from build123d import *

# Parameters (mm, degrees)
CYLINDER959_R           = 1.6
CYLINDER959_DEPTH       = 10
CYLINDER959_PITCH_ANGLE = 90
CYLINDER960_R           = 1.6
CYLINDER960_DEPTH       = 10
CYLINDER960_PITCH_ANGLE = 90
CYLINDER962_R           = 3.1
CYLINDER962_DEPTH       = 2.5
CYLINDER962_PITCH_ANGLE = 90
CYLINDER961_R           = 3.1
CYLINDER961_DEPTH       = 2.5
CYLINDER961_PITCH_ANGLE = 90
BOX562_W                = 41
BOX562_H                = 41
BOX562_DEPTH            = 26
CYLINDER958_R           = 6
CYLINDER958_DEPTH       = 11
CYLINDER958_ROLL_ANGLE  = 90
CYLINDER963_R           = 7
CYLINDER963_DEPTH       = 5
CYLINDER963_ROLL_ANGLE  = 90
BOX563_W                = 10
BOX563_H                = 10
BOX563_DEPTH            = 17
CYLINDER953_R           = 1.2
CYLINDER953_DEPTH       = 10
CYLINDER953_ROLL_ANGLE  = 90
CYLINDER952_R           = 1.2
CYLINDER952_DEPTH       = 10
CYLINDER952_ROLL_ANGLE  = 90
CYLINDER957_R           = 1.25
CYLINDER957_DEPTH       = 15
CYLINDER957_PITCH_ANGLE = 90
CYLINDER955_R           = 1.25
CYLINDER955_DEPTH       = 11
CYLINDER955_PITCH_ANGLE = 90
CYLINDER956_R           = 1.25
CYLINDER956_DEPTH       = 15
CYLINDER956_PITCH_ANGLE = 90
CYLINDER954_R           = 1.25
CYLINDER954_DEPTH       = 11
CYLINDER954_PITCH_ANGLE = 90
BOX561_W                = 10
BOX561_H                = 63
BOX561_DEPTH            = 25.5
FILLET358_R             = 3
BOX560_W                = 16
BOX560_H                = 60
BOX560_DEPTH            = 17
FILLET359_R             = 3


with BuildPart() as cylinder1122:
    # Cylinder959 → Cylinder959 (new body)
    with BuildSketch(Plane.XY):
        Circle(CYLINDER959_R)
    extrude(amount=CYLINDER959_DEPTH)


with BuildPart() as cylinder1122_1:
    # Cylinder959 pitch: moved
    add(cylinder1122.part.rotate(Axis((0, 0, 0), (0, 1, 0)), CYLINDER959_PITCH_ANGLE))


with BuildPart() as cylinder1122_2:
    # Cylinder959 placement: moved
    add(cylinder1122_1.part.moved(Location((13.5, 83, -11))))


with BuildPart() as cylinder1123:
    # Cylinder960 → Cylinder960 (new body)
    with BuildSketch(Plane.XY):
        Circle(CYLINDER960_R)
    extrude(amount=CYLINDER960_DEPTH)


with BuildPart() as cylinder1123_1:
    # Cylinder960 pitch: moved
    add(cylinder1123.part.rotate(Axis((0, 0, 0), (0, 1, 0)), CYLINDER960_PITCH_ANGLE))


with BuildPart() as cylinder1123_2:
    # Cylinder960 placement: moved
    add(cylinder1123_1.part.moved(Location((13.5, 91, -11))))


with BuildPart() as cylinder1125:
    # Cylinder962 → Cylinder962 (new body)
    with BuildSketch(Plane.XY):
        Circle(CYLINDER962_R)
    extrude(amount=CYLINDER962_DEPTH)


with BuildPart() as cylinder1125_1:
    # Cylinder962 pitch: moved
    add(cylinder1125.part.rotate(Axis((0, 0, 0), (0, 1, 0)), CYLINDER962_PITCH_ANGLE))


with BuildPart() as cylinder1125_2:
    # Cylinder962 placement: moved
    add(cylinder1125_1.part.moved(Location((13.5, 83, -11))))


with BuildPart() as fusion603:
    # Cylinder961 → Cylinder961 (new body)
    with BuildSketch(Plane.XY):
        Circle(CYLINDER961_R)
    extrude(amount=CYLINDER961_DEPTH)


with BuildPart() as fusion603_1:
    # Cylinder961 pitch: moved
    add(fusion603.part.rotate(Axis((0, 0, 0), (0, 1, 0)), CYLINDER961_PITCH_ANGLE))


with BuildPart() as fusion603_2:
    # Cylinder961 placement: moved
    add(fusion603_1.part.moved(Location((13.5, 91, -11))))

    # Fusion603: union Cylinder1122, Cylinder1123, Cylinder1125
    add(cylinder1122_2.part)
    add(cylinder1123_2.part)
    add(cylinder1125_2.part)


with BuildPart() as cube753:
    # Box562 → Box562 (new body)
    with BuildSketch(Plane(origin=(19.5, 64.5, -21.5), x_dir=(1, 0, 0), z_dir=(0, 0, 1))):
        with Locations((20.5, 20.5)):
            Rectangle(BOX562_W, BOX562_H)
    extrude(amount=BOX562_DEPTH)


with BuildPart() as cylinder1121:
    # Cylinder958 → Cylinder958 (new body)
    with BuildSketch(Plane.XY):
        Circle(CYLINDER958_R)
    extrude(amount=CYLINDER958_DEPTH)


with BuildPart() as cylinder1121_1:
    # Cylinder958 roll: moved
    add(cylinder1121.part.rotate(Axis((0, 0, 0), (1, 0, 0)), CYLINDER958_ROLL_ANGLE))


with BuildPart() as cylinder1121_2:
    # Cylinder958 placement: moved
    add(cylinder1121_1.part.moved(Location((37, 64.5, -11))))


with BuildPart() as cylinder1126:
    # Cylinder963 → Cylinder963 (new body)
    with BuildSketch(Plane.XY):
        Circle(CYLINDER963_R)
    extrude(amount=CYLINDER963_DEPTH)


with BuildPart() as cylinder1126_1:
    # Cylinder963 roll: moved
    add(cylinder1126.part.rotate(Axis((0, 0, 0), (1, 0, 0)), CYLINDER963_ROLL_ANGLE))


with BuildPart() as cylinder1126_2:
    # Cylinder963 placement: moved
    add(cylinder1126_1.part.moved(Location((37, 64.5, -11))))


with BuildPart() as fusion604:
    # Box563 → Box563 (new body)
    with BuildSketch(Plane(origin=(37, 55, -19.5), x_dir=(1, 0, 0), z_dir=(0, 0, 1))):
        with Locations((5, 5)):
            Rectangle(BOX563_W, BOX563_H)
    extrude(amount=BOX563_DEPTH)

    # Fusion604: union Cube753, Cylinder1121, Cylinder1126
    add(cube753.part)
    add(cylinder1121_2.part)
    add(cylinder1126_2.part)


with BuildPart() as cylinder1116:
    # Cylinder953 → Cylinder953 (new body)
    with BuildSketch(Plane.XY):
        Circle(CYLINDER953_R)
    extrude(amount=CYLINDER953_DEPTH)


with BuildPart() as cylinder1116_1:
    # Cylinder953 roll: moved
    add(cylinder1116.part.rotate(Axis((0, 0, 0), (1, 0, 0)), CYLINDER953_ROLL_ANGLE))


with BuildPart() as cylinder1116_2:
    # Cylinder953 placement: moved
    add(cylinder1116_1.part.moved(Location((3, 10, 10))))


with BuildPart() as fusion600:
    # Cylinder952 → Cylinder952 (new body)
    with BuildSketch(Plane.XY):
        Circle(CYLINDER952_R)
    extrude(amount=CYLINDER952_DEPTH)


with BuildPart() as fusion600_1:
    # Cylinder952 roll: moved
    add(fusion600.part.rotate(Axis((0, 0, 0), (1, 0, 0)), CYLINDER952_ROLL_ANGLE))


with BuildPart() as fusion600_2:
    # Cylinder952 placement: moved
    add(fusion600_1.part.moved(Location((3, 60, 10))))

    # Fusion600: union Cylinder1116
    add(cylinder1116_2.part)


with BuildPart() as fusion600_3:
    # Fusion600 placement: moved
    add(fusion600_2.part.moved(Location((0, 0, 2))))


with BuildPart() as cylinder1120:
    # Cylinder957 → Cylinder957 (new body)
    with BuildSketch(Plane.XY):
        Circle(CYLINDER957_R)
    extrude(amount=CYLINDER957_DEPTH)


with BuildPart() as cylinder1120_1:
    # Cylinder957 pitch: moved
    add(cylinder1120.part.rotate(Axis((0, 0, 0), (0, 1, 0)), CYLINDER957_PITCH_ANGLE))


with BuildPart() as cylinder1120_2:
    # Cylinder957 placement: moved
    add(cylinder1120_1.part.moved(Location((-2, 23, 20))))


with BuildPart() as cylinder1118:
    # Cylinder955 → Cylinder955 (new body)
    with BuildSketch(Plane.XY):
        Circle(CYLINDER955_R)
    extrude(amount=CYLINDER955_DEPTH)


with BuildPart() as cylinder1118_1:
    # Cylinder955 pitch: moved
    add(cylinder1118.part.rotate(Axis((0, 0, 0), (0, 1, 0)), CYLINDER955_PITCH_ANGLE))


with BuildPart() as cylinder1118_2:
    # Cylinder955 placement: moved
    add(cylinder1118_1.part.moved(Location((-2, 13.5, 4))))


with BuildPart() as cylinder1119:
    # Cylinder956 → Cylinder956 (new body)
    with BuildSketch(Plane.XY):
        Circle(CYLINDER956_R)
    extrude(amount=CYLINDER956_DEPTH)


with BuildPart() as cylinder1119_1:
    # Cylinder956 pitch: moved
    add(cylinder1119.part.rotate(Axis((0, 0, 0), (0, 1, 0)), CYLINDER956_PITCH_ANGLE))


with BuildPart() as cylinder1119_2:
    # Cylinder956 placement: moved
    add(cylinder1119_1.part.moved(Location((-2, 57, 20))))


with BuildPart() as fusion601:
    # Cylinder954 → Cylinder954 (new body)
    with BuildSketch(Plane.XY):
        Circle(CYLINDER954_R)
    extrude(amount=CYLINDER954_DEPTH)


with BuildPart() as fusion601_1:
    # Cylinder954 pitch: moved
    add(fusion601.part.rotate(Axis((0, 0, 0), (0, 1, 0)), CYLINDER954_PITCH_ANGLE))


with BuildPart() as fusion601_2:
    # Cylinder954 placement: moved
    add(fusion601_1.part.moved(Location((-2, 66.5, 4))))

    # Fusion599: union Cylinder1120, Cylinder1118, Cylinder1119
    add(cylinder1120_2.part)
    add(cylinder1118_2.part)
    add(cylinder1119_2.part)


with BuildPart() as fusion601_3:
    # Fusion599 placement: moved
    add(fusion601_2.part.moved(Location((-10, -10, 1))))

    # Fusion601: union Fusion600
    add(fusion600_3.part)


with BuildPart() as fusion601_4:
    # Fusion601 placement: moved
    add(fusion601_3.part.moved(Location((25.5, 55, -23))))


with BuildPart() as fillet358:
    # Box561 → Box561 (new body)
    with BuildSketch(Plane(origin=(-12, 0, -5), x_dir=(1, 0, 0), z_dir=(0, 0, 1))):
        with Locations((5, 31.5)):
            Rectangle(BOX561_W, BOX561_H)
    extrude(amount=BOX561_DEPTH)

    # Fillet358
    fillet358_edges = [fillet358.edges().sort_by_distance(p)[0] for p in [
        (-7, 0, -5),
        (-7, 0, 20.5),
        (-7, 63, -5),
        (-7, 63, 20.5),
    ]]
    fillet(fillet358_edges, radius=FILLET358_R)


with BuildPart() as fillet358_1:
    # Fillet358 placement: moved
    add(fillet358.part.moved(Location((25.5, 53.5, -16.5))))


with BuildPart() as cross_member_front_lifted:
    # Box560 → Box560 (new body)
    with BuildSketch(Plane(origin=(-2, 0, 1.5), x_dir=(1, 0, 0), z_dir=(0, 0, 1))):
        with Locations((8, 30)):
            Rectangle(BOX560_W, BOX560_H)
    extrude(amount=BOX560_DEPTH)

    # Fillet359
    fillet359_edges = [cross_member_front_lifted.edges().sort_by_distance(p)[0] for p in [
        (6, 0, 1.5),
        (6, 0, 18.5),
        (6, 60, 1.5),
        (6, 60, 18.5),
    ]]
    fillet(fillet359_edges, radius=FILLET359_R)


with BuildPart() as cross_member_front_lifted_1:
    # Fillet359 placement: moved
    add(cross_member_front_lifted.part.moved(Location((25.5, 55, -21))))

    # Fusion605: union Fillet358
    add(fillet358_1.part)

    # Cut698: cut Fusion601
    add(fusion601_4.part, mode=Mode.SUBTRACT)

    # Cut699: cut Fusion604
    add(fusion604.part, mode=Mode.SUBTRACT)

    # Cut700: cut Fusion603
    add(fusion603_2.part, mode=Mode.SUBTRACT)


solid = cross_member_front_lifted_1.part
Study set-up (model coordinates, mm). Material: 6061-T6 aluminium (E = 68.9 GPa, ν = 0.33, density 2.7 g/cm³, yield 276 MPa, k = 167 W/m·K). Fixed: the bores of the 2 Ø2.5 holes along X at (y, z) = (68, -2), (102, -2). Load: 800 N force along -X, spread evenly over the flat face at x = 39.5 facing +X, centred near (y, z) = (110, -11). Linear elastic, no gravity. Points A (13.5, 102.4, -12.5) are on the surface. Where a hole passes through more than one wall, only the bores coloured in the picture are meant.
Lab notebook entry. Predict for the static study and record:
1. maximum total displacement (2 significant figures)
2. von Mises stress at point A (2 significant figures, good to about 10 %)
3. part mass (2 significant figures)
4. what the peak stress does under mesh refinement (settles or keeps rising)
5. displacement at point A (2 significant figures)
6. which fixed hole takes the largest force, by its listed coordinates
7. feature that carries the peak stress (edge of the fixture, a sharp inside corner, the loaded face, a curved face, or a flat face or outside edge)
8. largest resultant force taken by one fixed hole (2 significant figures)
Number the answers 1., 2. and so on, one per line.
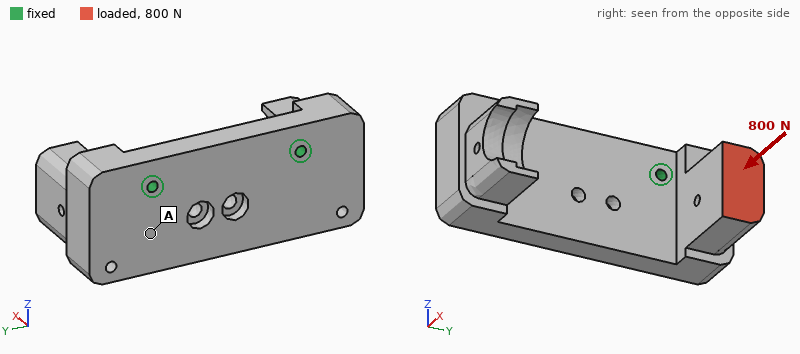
1. 75 µm
2. 19 MPa
3. 41 g
4. keeps rising
5. 19 µm
6. (102, -2)
7. edge of the fixture
8. 870 N
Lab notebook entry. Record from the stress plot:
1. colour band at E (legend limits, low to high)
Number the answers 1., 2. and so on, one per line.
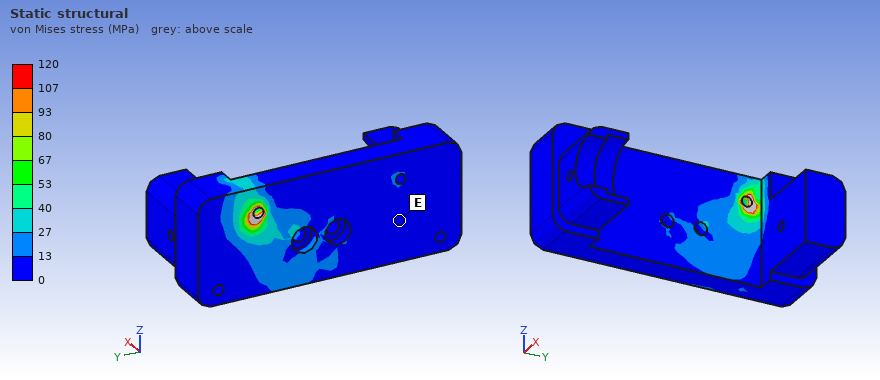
1. 0 to 13 MPa
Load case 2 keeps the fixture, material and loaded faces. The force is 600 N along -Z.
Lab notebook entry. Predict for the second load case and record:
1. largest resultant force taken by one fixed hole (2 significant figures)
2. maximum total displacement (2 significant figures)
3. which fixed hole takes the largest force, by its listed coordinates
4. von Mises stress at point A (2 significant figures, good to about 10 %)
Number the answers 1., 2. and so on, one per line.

1. 730 N
2. 0.11 mm
3. (102, -2)
4. 23 MPa
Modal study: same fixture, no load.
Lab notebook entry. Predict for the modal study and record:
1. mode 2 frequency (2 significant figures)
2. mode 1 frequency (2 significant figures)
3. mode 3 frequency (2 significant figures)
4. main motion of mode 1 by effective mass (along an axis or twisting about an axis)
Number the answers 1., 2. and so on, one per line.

1. 5800 Hz
2. 4700 Hz
3. 6300 Hz
4. along X
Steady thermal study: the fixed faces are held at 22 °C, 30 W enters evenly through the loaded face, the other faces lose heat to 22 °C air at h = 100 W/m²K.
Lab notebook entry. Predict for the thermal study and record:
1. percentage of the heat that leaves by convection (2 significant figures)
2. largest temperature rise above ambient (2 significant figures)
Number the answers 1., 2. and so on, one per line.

1. 15 %
2. 35 K
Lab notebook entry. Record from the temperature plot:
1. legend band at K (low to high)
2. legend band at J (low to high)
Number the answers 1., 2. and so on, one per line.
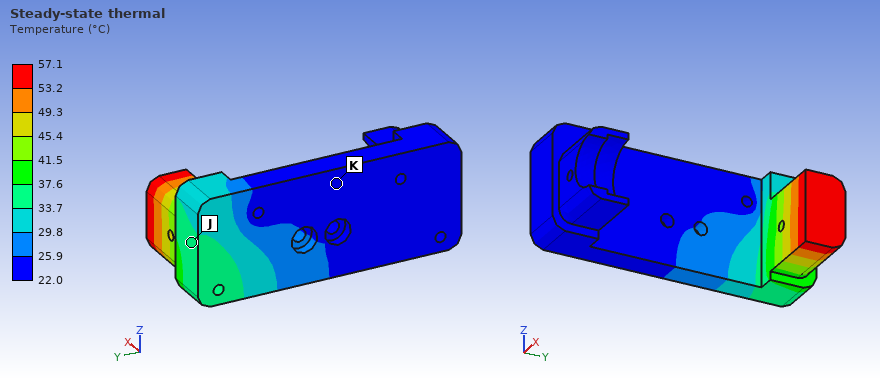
1. 22.0 to 25.9 °C
2. 33.7 to 37.6 °C
